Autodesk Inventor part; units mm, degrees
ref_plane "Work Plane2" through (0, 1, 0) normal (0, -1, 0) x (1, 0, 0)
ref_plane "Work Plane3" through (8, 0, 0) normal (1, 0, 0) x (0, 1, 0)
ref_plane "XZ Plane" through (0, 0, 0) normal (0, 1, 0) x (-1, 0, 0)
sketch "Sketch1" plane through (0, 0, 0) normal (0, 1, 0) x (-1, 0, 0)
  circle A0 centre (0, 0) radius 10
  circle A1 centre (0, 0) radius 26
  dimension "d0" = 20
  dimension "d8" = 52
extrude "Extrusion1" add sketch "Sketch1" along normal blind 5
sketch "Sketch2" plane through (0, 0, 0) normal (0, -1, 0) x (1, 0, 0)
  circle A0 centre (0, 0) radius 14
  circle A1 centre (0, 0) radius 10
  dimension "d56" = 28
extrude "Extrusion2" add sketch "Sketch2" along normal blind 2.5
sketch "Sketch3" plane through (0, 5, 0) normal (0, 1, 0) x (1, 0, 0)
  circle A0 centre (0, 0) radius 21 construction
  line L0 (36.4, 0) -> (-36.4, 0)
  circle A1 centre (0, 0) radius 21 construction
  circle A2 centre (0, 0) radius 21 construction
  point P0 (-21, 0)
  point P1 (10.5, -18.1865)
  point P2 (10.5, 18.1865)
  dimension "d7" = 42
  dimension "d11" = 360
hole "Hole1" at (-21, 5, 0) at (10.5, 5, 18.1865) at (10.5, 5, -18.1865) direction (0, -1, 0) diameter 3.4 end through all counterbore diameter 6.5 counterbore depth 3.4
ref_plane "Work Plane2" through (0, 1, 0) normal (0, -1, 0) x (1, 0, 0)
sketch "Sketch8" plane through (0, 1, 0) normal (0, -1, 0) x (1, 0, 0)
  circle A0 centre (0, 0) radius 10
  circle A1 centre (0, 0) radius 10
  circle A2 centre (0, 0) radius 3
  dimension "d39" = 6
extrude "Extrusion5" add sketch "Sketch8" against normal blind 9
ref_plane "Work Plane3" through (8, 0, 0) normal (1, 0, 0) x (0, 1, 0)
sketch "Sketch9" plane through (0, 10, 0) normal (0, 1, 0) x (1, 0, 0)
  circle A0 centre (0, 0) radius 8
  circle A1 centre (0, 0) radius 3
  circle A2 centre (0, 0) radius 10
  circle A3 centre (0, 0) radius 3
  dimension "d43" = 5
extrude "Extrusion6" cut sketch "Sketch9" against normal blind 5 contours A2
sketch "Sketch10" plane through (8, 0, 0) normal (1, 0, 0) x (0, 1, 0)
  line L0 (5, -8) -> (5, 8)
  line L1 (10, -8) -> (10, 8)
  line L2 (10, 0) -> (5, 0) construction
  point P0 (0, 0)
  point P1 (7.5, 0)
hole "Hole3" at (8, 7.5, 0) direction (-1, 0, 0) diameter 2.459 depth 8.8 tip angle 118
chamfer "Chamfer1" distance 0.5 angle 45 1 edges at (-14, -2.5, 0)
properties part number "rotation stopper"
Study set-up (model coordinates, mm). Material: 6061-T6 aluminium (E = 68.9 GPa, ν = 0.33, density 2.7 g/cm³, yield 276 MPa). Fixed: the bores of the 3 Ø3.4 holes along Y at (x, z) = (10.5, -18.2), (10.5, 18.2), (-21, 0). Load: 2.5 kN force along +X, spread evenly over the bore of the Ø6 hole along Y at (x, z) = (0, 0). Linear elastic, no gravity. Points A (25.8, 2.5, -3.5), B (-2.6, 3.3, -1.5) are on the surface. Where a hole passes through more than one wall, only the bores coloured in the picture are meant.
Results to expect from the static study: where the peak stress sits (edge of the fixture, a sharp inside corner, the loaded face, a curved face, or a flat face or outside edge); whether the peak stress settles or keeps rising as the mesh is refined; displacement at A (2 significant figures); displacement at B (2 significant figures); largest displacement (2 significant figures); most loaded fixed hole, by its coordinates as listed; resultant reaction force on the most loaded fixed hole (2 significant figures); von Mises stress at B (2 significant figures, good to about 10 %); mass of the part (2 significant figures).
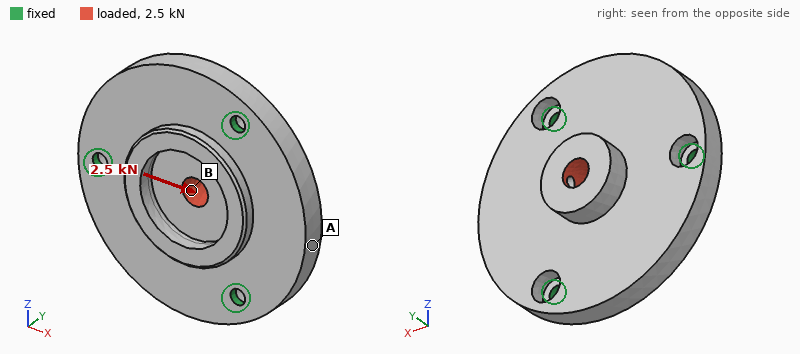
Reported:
edge of the fixture
keeps rising
20 µm
7.4 µm
21 µm
(-21, 0)
1.1 kN
21 MPa
31 g
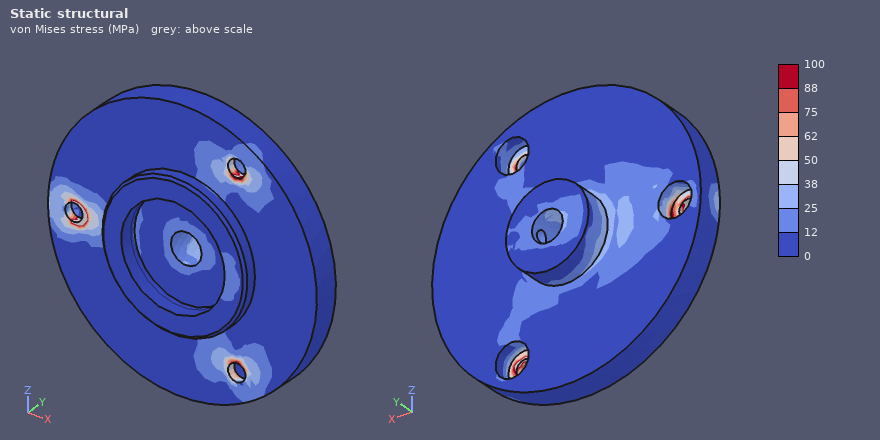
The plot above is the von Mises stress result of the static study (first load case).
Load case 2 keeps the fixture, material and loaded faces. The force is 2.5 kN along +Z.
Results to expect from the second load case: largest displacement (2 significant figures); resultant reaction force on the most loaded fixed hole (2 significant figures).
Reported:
19 µm
1.0 kN
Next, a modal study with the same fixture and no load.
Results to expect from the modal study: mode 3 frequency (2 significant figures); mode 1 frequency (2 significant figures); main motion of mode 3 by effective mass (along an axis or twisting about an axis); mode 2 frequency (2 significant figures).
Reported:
10 kHz
8900 Hz
along Y
8900 Hz
